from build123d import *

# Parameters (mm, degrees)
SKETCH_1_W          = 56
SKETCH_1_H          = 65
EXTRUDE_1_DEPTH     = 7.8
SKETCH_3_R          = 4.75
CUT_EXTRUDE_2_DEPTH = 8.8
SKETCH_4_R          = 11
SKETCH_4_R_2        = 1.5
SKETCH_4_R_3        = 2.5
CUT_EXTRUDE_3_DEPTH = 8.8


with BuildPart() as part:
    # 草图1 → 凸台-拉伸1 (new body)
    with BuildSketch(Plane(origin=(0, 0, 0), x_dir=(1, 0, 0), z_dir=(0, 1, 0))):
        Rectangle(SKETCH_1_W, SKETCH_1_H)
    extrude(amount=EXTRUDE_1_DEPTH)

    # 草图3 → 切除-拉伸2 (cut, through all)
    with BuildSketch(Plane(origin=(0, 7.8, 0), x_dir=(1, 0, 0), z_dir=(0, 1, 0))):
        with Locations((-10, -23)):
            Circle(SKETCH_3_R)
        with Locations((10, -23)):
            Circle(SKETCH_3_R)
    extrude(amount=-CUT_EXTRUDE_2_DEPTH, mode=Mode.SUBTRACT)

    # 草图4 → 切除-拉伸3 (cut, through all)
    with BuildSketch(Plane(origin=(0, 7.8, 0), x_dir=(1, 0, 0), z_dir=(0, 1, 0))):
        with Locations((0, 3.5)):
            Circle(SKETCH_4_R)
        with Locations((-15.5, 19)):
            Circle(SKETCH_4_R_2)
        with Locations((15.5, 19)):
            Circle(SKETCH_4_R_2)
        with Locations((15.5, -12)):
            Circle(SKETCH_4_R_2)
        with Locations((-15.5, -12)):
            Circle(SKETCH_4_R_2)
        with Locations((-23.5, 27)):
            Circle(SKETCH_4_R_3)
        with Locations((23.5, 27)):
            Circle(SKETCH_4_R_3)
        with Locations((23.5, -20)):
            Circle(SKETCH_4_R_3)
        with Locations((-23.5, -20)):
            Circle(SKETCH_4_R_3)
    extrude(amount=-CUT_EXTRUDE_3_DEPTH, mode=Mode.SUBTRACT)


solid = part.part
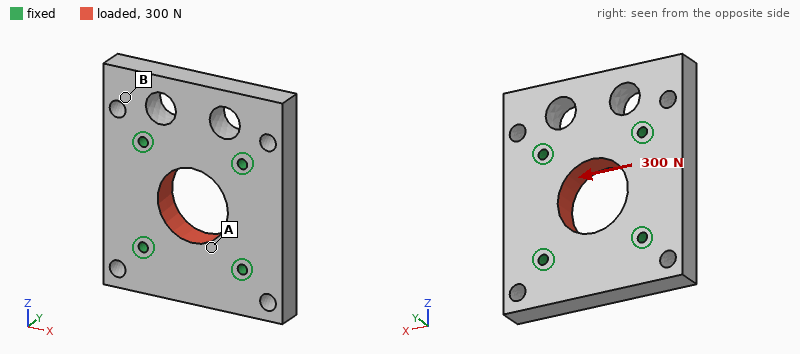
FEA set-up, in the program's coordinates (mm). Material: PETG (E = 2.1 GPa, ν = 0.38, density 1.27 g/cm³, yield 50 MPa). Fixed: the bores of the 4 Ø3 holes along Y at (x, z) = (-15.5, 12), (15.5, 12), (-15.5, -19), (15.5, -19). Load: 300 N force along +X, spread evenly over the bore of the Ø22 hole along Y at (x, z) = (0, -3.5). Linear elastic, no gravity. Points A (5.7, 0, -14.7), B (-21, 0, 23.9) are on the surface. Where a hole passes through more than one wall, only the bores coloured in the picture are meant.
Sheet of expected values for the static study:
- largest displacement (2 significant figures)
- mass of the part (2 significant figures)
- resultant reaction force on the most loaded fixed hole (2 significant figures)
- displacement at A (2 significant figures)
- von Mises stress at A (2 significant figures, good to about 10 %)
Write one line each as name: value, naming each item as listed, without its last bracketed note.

largest displacement: 8.2 µm
mass of the part: 30 g
resultant reaction force on the most loaded fixed hole: 76 N
displacement at A: 4.2 µm
von Mises stress at A: 0.86 MPa
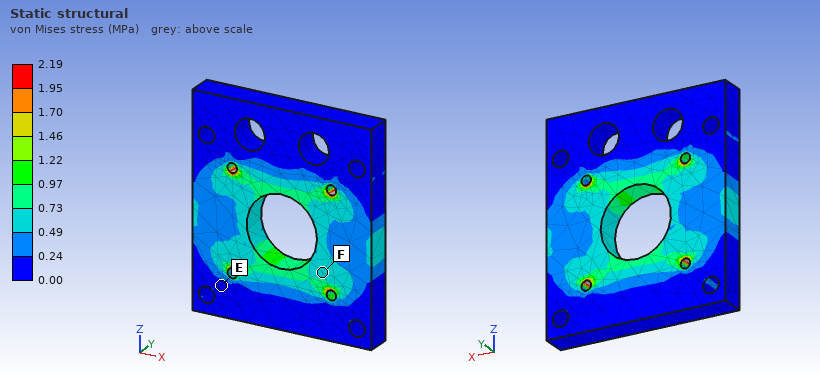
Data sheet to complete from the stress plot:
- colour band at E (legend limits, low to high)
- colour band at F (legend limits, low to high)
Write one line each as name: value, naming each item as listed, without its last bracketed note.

colour band at E: 0.00 to 0.24 MPa
colour band at F: 0.49 to 0.73 MPa
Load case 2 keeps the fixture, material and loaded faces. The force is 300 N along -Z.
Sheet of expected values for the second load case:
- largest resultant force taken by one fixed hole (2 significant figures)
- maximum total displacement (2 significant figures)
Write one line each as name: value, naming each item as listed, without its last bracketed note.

largest resultant force taken by one fixed hole: 77 N
maximum total displacement: 8.7 µm
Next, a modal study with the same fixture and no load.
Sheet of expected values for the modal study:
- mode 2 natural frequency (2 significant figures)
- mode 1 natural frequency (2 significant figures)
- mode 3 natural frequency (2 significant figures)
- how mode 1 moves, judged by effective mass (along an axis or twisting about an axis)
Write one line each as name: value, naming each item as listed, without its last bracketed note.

mode 2 natural frequency: 3300 Hz
mode 1 natural frequency: 2600 Hz
mode 3 natural frequency: 4500 Hz
how mode 1 moves, judged by effective mass: along Y
